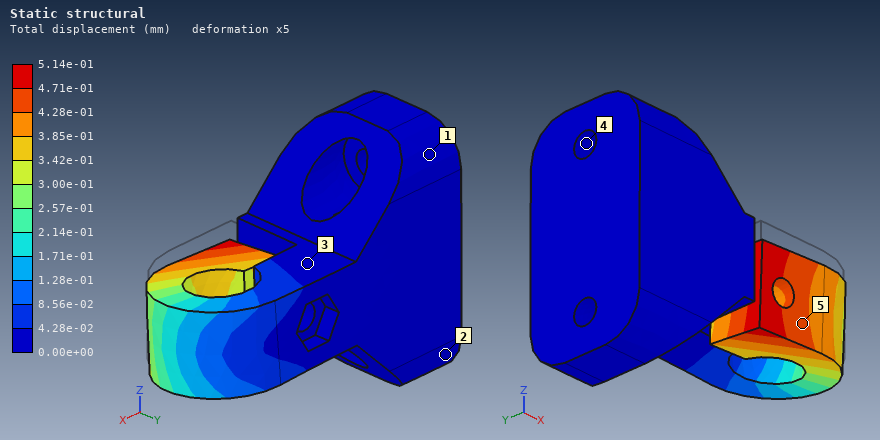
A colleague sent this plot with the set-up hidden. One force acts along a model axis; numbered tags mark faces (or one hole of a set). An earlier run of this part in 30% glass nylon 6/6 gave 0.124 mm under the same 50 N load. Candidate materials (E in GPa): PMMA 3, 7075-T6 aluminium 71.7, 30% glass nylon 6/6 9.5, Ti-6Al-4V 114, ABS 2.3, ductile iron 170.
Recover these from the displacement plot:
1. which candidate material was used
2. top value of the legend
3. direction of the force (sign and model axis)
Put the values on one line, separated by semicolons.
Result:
ABS; 5.14e-01 mm; -Z
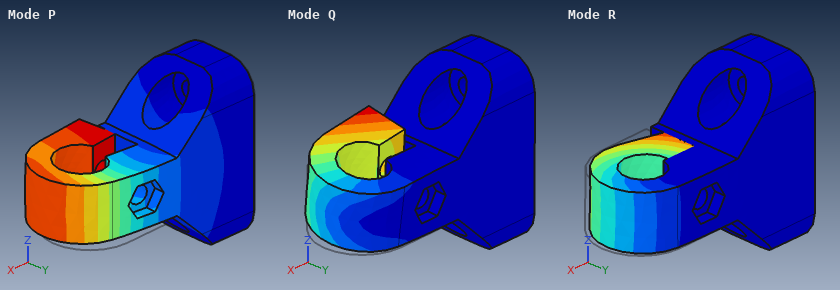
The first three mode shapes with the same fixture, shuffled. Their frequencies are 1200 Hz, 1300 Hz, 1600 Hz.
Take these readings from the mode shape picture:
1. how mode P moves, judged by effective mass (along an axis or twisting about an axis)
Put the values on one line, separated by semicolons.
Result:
along Y
